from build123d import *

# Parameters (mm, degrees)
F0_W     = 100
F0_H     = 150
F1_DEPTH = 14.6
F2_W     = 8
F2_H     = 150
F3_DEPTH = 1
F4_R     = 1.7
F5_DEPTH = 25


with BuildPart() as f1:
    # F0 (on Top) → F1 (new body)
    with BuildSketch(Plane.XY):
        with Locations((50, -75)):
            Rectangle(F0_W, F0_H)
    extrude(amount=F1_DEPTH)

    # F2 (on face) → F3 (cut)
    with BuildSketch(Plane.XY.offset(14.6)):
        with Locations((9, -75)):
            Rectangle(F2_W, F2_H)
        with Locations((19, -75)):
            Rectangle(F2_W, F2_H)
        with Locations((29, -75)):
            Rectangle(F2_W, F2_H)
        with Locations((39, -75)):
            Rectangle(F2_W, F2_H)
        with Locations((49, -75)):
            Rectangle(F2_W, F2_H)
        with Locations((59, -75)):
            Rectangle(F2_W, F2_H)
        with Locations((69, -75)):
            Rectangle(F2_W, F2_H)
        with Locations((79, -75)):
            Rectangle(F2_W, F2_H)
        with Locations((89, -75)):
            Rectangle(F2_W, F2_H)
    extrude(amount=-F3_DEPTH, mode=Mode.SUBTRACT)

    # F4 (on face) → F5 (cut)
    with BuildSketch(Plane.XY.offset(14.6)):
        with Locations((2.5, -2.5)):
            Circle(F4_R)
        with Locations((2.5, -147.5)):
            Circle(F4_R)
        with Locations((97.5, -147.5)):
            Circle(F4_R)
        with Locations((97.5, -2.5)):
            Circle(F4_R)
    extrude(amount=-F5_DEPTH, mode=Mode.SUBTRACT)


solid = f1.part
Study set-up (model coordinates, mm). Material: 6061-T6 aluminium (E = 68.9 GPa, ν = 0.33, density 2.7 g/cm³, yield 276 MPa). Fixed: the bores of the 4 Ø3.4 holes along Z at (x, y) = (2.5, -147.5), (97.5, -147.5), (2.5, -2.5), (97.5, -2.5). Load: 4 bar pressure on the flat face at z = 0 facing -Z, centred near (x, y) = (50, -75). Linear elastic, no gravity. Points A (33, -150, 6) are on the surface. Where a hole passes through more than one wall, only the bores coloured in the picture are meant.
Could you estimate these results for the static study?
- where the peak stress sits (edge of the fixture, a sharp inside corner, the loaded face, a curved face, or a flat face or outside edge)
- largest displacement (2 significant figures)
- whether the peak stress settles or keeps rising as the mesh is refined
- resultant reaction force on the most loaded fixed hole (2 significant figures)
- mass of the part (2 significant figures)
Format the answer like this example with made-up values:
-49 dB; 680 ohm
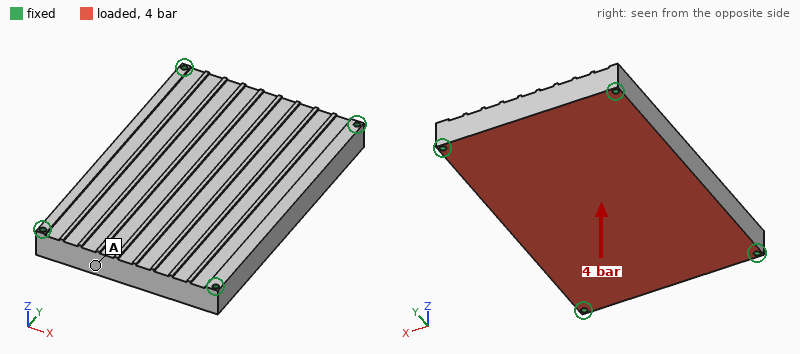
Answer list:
edge of the fixture; 73 µm; keeps rising; 1.5 kN; 560 g
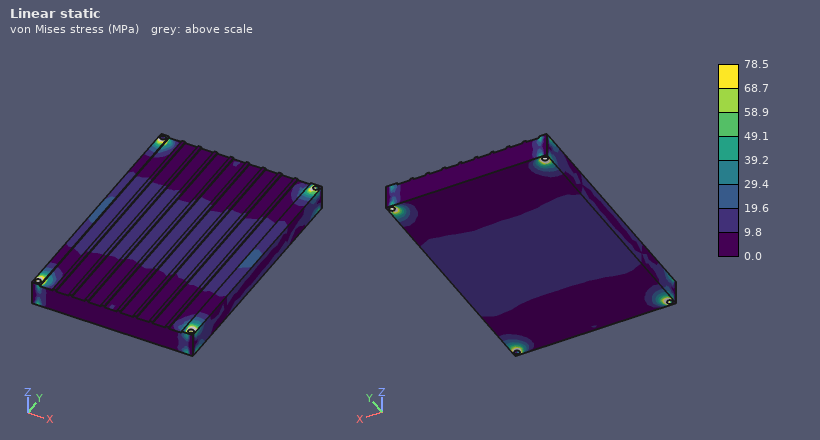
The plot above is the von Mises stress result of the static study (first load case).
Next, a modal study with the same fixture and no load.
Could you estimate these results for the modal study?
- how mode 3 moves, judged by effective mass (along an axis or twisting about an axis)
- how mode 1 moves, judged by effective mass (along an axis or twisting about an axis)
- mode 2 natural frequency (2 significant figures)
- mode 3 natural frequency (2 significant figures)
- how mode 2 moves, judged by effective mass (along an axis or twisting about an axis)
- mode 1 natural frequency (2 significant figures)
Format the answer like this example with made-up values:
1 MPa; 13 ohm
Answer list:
twisting about X; along Z; 3800 Hz; 5200 Hz; twisting about Y; 2200 Hz
